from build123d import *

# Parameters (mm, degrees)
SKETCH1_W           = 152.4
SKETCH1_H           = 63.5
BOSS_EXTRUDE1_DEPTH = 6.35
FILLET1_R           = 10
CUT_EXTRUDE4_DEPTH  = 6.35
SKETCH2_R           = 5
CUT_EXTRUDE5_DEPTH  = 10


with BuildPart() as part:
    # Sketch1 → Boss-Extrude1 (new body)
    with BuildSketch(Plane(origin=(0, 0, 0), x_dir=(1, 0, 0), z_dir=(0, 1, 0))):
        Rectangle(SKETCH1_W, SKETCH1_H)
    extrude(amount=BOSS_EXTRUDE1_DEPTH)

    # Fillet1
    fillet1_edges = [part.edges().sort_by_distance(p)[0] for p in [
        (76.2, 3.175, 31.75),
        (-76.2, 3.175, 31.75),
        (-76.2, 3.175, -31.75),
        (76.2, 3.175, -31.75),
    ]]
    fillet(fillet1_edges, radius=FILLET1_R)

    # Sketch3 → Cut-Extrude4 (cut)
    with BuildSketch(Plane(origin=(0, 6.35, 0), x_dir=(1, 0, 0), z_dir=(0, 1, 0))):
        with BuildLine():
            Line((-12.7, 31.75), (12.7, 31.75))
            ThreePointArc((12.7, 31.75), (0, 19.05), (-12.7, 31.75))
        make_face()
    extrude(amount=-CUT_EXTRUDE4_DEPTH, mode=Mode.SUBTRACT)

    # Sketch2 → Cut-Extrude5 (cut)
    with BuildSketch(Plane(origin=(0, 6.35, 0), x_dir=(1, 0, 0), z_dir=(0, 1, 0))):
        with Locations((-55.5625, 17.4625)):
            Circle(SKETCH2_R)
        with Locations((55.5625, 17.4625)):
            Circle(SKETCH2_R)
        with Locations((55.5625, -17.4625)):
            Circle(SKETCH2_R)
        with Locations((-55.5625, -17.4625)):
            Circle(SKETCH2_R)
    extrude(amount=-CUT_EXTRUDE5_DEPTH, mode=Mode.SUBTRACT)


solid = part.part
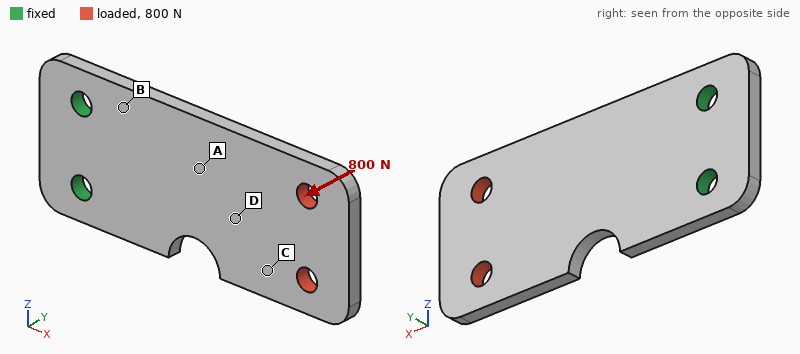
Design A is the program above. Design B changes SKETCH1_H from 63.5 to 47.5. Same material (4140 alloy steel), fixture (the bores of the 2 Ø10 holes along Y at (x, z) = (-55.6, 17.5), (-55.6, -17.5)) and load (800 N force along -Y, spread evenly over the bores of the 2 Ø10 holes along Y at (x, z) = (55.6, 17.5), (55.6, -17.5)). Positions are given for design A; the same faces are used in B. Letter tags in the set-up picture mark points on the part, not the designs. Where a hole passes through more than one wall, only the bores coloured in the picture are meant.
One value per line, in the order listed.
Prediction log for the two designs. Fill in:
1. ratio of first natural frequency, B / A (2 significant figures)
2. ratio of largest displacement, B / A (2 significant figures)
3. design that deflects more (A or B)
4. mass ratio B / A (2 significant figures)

1.0
1.3
B
0.75
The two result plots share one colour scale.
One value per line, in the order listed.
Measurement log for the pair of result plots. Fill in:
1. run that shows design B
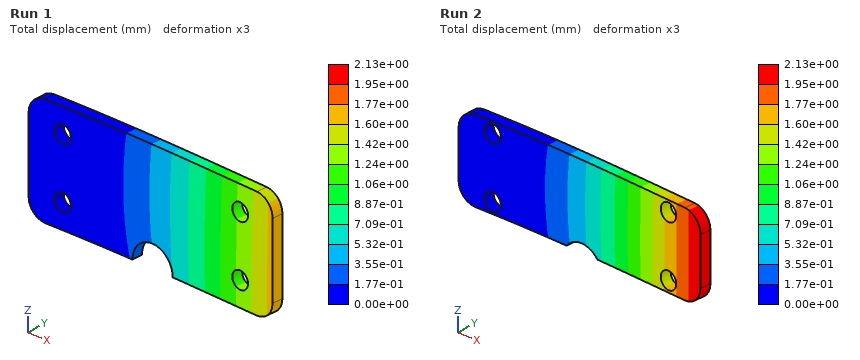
Run 2
